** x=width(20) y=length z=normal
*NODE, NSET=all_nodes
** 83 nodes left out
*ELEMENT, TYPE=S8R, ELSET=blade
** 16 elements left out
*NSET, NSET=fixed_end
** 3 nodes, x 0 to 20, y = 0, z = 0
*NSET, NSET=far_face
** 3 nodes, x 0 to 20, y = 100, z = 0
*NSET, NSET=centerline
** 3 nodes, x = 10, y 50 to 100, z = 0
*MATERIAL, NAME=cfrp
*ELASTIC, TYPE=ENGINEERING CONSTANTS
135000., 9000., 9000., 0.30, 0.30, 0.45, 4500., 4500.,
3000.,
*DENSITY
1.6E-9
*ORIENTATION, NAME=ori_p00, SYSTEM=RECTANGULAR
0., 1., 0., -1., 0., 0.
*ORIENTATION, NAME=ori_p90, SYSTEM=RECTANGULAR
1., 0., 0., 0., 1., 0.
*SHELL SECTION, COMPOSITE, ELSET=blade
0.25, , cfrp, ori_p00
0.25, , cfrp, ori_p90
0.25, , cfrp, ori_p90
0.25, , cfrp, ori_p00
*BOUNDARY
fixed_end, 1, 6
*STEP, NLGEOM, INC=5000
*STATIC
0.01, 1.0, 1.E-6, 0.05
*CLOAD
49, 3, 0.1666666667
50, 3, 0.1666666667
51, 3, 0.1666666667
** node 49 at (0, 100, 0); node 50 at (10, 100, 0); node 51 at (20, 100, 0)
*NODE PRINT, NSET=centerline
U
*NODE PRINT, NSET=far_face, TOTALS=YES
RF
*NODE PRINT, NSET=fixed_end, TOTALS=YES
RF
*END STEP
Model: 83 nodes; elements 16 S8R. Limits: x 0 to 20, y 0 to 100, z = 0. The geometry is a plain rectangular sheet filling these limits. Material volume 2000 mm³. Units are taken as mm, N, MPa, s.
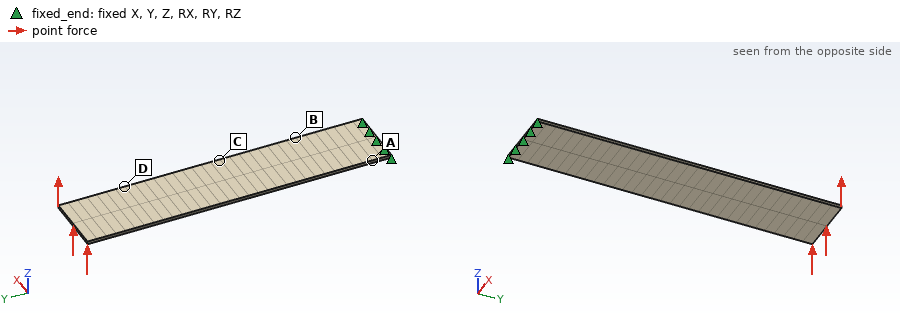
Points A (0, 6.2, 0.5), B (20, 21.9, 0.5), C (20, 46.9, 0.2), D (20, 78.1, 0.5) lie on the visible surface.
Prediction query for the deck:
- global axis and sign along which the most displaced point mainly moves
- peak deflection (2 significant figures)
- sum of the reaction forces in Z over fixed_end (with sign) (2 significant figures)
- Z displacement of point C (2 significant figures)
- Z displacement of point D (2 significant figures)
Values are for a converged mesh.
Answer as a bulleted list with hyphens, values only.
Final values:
- +Z
- 0.84 mm
- -0.50 N
- 0.23 mm
- 0.57 mm
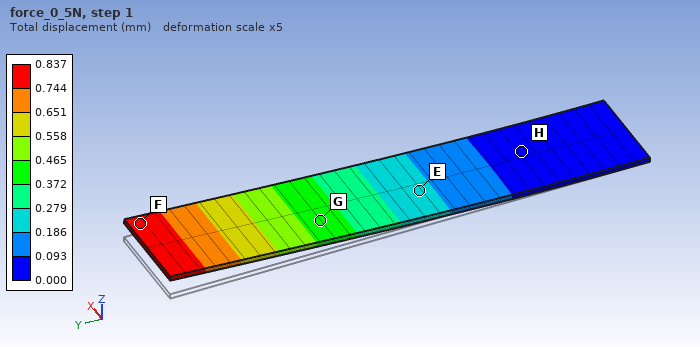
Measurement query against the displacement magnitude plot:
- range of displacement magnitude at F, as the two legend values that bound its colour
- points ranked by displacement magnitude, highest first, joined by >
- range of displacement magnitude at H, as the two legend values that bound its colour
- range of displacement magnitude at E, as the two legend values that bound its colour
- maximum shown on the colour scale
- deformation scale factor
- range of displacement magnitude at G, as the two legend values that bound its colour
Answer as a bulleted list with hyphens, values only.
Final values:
- 0.744 to 0.837 mm
- F > G > E > H
- 0.000 to 0.093 mm
- 0.186 to 0.279 mm
- 0.837 mm
- 5
- 0.372 to 0.465 mm
